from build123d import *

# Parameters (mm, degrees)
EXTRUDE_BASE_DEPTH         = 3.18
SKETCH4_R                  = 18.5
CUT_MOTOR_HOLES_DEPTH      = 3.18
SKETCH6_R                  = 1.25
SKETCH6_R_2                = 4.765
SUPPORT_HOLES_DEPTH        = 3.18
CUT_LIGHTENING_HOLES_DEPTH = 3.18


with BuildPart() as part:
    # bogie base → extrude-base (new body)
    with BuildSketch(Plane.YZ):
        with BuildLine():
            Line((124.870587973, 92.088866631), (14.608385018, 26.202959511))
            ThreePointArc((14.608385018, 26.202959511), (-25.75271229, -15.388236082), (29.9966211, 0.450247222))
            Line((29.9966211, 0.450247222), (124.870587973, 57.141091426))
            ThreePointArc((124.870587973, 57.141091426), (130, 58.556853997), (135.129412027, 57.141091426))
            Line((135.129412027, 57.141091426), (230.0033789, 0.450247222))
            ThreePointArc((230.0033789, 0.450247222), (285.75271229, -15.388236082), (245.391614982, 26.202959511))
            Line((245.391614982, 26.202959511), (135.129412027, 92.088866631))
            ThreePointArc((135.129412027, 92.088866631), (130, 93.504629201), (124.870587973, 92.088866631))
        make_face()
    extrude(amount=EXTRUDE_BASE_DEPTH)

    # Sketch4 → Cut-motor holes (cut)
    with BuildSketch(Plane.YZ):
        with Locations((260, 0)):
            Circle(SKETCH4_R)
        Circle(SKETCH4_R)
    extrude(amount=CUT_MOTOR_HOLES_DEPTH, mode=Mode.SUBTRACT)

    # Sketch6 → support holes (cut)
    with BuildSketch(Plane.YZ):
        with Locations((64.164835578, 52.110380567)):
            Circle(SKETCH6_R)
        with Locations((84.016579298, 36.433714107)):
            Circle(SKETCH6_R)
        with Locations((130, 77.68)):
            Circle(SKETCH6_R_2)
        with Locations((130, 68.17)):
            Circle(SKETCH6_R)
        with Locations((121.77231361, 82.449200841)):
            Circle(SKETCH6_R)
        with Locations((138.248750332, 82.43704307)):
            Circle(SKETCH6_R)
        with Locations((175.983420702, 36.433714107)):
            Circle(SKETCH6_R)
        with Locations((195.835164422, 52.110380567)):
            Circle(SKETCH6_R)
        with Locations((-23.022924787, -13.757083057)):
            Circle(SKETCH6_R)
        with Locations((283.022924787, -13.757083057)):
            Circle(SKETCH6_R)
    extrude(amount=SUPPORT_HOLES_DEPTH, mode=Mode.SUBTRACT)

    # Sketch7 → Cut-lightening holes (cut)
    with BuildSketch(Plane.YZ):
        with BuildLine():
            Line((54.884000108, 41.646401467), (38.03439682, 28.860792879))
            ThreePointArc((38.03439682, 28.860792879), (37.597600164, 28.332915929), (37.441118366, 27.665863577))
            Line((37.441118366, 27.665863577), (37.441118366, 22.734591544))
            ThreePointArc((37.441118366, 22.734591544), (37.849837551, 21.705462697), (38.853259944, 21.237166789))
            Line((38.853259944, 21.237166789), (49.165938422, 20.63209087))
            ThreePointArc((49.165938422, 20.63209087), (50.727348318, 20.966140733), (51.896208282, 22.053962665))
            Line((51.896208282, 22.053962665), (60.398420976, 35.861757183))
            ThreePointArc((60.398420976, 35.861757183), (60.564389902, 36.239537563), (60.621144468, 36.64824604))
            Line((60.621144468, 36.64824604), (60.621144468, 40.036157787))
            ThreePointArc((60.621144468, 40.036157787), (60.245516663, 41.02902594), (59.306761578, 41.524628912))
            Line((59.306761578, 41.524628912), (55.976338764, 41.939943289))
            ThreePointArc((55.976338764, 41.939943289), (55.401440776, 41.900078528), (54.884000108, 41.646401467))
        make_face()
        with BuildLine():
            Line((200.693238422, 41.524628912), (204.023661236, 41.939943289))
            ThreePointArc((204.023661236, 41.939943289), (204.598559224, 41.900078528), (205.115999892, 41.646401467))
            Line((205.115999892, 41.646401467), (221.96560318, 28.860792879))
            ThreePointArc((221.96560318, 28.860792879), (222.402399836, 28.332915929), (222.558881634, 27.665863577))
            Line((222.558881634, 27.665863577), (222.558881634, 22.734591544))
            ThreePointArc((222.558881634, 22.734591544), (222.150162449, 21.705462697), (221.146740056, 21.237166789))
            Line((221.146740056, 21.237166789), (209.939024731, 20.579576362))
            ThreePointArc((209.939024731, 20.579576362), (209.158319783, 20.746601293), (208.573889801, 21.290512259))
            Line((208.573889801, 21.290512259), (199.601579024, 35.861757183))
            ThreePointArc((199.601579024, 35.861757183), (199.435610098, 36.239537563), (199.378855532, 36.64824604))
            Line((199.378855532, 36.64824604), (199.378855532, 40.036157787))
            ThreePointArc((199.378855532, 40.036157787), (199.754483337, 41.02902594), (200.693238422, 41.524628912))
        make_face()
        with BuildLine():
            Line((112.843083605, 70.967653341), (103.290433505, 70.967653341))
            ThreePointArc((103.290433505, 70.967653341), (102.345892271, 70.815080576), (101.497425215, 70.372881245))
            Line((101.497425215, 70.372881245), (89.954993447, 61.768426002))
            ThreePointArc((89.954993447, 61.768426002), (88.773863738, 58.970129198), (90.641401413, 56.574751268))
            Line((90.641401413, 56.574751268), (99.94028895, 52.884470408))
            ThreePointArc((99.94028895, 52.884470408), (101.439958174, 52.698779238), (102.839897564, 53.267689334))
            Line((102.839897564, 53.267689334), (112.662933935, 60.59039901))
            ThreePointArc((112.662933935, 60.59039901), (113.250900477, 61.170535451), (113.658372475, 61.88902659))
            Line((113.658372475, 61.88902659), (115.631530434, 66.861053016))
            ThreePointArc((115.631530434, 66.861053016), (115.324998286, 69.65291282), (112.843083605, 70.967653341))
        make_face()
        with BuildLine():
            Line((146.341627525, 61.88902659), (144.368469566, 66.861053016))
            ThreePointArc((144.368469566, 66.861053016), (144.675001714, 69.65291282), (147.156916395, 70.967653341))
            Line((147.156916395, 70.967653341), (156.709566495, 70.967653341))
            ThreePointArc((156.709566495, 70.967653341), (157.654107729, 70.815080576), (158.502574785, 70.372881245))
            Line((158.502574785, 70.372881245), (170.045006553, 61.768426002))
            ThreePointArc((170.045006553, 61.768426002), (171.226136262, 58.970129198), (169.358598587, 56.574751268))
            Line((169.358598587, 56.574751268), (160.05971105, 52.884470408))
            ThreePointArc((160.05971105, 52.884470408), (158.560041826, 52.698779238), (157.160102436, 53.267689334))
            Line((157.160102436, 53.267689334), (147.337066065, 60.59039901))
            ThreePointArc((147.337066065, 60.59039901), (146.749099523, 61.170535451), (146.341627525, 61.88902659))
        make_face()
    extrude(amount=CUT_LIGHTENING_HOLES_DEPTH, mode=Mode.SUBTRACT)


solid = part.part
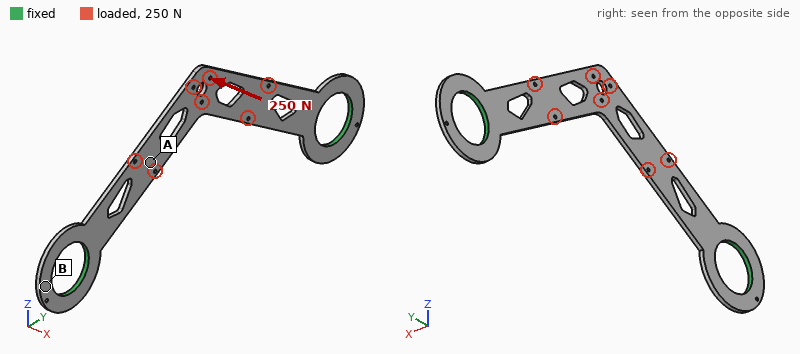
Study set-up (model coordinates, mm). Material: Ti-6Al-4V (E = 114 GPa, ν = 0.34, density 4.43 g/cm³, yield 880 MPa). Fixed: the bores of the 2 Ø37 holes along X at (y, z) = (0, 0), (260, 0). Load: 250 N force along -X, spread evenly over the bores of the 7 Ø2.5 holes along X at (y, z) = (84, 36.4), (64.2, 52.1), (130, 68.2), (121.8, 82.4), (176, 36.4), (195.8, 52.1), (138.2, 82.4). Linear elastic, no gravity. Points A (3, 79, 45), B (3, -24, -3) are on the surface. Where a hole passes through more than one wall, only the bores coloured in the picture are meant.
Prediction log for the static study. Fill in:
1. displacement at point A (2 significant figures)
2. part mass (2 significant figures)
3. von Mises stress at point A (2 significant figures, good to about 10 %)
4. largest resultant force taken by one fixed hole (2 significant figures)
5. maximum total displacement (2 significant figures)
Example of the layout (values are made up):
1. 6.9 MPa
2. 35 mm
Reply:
1. 1.7 mm
2. 130 g
3. 40 MPa
4. 130 N
5. 4.0 mm
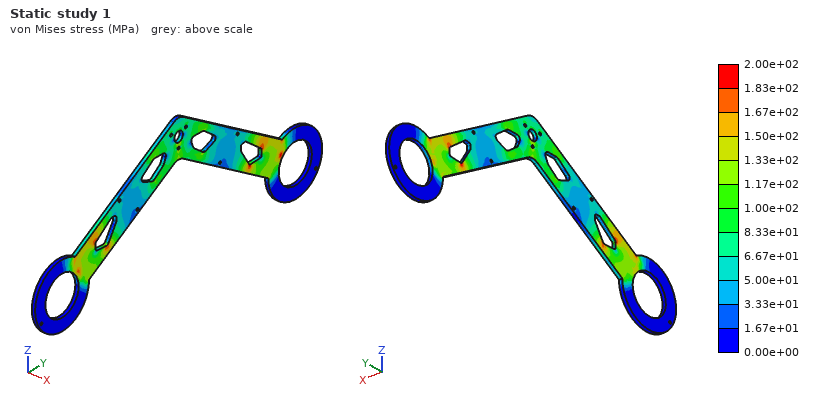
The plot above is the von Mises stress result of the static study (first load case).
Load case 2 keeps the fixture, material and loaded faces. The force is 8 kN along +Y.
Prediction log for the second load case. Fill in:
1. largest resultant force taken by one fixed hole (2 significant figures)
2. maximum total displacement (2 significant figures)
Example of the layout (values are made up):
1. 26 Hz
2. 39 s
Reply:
1. 4.3 kN
2. 0.11 mm
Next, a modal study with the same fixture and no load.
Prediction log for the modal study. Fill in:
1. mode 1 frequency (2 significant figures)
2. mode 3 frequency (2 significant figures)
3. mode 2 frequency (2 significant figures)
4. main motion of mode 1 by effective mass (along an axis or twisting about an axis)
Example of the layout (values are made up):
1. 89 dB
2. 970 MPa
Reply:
1. 210 Hz
2. 930 Hz
3. 670 Hz
4. along X
